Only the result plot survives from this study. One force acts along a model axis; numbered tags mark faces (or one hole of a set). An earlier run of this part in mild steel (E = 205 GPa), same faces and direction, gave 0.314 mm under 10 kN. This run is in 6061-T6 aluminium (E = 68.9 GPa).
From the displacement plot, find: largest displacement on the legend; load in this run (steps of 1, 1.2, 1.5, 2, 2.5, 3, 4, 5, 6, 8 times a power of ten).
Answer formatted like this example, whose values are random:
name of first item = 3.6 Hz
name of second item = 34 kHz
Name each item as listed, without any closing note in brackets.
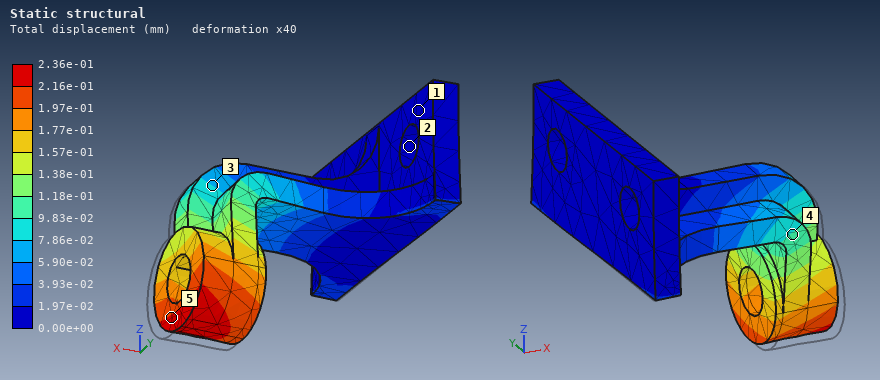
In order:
largest displacement on the legend = 2.36e-01 mm
load in this run = 2.5 kN
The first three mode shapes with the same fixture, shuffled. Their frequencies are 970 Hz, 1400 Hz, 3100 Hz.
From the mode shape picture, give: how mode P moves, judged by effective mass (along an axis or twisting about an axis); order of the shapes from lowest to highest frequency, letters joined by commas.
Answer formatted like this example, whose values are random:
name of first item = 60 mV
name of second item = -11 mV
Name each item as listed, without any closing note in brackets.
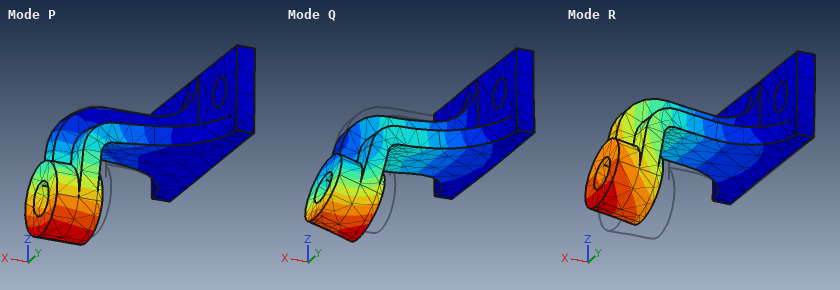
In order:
how mode P moves, judged by effective mass = along Y
order of the shapes from lowest to highest frequency, letters joined by commas = R, P, Q
